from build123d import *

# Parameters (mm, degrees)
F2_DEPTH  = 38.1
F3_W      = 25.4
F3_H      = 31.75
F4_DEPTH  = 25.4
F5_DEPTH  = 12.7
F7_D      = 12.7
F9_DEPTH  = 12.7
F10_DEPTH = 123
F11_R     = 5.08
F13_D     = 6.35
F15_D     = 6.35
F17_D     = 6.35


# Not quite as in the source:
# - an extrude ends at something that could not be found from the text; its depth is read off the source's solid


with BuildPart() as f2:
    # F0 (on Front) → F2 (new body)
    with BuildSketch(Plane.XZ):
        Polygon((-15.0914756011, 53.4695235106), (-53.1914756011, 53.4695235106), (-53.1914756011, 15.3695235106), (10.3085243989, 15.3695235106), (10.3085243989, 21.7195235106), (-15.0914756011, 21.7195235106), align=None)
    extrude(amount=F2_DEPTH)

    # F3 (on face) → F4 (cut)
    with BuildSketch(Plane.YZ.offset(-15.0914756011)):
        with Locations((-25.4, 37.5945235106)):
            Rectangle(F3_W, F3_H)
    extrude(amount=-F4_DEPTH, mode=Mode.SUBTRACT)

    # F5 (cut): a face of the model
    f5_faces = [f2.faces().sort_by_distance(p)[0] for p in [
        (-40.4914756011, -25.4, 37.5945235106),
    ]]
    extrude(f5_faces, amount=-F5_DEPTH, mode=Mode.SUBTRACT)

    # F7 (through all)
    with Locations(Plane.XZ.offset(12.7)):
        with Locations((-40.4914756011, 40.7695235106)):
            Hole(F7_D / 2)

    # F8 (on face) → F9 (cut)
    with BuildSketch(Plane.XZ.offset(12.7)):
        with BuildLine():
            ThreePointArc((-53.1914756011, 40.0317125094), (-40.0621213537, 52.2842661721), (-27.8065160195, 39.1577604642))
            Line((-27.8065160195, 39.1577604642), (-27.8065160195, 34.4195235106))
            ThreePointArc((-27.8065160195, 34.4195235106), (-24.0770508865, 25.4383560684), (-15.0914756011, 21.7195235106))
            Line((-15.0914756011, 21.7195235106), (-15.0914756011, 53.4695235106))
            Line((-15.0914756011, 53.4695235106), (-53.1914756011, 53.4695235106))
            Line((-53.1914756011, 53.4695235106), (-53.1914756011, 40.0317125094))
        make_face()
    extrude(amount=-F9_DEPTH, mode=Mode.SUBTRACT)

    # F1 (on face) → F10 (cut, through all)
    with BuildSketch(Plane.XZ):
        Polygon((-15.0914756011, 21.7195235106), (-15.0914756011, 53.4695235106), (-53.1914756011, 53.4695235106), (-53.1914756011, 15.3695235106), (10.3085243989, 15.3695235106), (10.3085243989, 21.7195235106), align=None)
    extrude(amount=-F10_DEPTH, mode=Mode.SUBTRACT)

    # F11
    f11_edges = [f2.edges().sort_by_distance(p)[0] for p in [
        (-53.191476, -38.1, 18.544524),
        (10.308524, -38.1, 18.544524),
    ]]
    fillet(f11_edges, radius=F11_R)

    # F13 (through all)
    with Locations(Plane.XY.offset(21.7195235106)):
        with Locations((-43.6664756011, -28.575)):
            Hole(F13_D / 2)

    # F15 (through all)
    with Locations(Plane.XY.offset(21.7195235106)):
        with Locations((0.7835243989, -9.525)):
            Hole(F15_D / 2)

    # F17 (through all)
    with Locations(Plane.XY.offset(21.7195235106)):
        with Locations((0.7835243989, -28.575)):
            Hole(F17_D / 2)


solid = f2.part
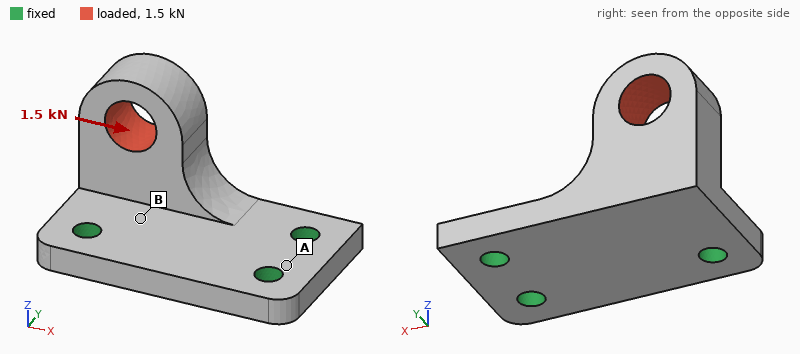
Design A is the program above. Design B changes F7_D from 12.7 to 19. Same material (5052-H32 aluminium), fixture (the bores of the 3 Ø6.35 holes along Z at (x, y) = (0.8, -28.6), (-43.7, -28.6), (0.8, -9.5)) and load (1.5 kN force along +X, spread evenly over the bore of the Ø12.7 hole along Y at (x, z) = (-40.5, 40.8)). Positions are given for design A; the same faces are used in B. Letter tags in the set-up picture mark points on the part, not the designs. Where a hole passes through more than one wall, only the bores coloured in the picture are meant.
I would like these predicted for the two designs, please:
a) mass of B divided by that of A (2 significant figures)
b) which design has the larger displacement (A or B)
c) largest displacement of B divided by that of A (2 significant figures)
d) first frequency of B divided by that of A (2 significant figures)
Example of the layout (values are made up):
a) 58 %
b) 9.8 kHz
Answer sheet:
a) 0.91
b) B
c) 1.4
d) 1.2
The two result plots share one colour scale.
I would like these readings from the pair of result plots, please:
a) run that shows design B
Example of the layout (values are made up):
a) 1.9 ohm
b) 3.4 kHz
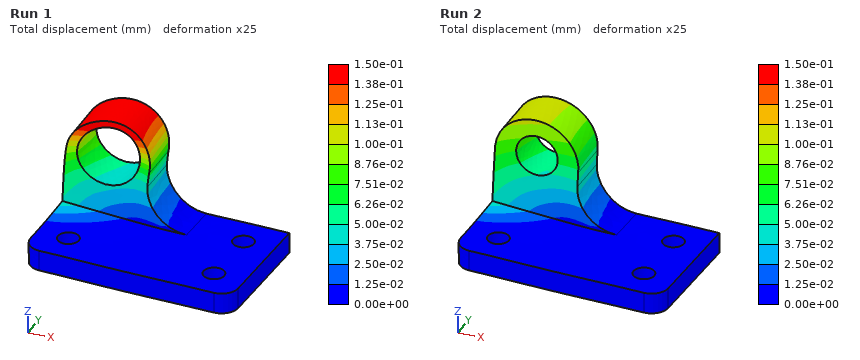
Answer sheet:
a) Run 1
